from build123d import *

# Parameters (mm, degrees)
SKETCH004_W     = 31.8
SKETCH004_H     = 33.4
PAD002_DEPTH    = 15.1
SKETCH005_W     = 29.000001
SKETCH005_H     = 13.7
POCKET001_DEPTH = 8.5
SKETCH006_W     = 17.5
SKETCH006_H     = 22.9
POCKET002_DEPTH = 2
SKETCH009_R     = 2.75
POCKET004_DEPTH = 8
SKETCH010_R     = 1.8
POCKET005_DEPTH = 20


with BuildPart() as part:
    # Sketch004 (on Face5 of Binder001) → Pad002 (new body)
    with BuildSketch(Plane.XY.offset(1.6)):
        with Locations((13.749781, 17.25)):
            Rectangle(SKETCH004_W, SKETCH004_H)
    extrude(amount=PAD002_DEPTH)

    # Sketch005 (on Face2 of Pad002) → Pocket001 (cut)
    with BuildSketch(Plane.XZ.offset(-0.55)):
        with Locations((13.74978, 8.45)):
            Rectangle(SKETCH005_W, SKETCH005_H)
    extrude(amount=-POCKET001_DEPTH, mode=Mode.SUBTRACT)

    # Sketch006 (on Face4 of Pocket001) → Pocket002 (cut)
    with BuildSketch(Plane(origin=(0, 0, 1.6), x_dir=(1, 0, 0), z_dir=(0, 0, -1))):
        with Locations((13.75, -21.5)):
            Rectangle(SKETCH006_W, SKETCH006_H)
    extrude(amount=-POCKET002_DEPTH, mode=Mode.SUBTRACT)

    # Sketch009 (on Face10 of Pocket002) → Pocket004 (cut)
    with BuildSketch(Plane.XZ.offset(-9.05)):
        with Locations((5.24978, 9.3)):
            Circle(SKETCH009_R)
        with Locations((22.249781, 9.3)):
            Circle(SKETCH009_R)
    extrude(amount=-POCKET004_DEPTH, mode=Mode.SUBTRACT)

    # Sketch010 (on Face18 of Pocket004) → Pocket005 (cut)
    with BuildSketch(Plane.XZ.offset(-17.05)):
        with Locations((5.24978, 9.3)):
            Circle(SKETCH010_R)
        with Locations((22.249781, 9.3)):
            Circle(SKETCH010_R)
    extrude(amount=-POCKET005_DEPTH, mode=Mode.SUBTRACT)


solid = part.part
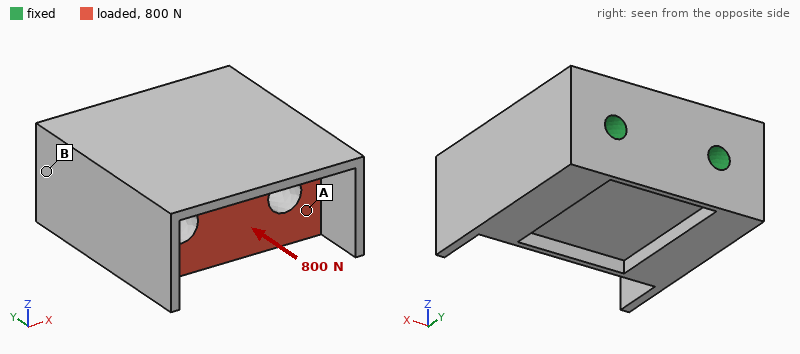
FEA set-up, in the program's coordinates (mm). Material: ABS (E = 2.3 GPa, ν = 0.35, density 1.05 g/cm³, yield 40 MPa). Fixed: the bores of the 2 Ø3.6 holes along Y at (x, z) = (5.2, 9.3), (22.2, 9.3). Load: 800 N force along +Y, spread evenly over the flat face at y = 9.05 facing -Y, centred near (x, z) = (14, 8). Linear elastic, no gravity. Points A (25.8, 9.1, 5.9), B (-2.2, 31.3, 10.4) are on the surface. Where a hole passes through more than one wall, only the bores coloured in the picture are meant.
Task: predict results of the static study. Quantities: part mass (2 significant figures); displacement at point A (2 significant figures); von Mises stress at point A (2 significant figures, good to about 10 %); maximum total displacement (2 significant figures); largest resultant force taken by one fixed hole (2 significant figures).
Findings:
12 g
19 µm
2.6 MPa
95 µm
410 N
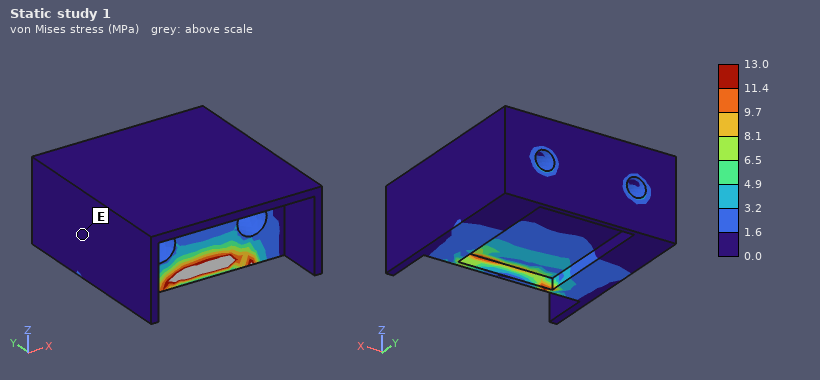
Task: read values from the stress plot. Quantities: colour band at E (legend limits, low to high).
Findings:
0.0 to 1.6 MPa
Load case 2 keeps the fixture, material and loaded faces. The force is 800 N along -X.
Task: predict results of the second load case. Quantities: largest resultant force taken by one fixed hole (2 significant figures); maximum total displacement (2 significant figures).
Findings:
560 N
0.11 mm
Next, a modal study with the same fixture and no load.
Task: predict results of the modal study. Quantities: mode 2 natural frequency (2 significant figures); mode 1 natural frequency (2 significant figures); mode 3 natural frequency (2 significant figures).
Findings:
5100 Hz
4800 Hz
5400 Hz
